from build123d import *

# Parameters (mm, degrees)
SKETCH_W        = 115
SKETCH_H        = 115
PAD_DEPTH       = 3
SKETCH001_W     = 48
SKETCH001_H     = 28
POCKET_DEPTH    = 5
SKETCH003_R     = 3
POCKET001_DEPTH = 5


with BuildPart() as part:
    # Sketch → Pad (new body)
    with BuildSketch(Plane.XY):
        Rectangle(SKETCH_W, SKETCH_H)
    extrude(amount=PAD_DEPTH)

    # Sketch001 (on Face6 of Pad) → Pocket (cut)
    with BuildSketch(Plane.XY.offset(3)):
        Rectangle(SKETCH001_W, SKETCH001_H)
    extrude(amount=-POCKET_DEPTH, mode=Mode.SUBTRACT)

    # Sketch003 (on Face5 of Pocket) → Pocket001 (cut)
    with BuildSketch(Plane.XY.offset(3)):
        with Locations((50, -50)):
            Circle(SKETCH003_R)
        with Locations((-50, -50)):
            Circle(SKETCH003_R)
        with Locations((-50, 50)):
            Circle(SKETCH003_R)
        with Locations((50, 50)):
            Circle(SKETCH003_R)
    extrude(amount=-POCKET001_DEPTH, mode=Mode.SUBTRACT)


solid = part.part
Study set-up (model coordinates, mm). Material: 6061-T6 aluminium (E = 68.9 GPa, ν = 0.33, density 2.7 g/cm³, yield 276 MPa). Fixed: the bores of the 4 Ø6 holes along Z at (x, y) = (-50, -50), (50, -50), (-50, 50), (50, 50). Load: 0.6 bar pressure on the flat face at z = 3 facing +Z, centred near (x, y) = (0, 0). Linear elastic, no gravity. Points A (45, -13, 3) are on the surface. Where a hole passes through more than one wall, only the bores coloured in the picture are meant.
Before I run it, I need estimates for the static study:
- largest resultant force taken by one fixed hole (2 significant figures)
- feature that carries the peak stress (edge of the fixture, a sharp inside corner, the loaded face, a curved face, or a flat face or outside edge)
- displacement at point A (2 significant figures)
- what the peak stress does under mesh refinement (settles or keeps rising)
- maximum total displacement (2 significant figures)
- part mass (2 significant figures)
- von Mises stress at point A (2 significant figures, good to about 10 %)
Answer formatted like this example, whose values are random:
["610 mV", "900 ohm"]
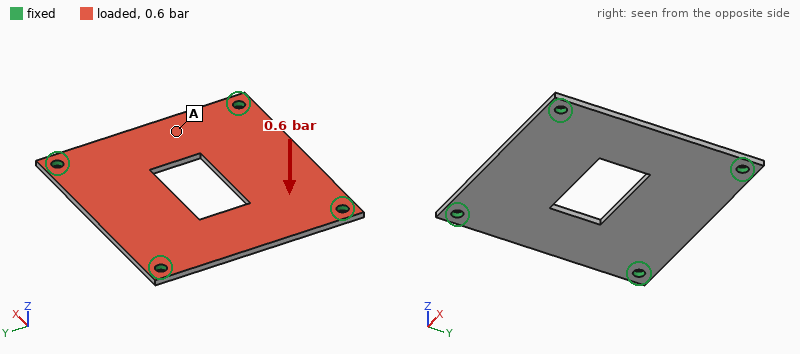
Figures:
["180 N", "edge of the fixture", "0.13 mm", "keeps rising", "0.28 mm", "95 g", "18 MPa"]
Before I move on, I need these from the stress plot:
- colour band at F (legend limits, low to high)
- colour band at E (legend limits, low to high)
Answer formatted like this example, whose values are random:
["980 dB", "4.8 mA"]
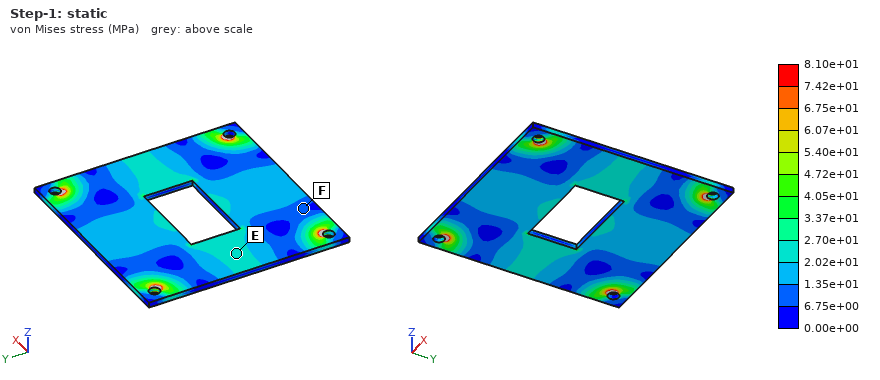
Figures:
["6.75e+00 to 1.35e+01 MPa", "2.02e+01 to 2.70e+01 MPa"]
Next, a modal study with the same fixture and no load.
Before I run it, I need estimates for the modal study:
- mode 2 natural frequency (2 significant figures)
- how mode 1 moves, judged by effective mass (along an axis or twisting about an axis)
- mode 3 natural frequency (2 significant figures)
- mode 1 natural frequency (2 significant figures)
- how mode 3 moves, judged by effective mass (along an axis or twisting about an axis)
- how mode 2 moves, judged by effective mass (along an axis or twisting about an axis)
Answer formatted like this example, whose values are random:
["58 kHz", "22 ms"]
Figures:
["1700 Hz", "along Z", "1800 Hz", "1100 Hz", "twisting about Y", "twisting about X"]
